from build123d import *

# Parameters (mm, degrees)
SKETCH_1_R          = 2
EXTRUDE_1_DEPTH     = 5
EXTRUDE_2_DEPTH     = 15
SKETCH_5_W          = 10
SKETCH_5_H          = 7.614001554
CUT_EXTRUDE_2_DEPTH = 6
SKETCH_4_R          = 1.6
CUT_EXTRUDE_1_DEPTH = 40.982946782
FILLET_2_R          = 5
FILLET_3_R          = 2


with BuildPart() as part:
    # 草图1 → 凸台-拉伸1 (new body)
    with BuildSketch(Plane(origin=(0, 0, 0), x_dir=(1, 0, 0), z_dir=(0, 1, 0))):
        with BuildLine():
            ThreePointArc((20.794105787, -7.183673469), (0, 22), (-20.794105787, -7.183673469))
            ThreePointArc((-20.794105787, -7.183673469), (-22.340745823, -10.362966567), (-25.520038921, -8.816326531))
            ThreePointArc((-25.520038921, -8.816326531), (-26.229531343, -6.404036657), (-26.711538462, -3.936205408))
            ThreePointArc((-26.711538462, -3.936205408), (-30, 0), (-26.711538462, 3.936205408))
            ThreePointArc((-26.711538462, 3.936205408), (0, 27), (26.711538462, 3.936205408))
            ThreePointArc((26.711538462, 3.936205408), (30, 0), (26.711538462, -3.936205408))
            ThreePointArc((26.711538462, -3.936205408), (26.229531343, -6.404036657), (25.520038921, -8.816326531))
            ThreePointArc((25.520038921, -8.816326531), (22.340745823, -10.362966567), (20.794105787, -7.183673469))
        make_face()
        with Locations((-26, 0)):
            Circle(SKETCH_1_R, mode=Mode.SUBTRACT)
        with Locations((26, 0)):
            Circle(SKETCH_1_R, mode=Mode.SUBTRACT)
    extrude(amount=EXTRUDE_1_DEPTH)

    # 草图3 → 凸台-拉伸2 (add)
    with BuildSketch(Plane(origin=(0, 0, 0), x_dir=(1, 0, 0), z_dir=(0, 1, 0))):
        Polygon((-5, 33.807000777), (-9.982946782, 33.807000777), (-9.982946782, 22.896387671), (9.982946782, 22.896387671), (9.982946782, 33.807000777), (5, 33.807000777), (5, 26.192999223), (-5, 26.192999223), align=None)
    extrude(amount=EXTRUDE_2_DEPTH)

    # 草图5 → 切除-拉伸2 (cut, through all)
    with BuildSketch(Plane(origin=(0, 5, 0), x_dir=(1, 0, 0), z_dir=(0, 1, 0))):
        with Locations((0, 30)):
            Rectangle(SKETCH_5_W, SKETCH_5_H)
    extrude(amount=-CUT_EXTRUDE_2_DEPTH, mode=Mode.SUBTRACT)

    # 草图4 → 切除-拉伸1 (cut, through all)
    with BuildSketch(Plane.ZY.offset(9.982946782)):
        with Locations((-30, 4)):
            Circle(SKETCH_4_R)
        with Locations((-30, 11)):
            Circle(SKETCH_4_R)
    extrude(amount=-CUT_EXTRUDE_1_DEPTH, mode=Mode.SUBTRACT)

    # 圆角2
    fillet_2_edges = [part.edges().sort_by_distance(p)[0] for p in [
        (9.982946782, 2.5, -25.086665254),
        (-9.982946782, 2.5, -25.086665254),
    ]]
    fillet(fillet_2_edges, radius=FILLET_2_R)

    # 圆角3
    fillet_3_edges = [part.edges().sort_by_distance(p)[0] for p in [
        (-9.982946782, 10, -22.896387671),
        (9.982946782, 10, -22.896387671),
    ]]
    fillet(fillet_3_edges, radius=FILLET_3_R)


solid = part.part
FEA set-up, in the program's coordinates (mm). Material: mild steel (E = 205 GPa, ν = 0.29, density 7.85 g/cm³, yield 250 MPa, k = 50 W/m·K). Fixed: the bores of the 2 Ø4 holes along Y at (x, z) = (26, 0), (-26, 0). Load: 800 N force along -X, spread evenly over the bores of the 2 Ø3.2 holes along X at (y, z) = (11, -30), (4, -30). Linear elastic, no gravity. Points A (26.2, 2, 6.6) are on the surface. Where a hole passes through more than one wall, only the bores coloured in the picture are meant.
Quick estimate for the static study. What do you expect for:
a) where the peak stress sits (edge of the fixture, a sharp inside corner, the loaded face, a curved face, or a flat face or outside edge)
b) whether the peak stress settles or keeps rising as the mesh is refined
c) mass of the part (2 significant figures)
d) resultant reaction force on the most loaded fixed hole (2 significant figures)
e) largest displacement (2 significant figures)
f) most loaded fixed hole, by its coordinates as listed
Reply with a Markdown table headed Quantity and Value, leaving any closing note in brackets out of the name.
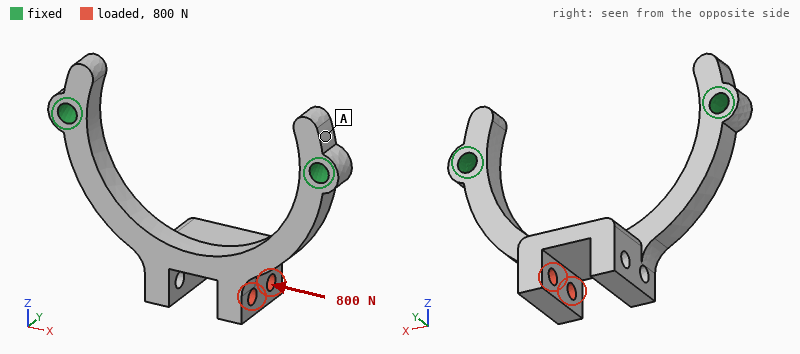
| Quantity | Value |
|---|---|
| where the peak stress sits | a sharp inside corner |
| whether the peak stress settles or keeps rising as the mesh is refined | keeps rising |
| mass of the part | 32 g |
| resultant reaction force on the most loaded fixed hole | 580 N |
| largest displacement | 38 µm |
| most loaded fixed hole, by its coordinates as listed | (-26, 0) |
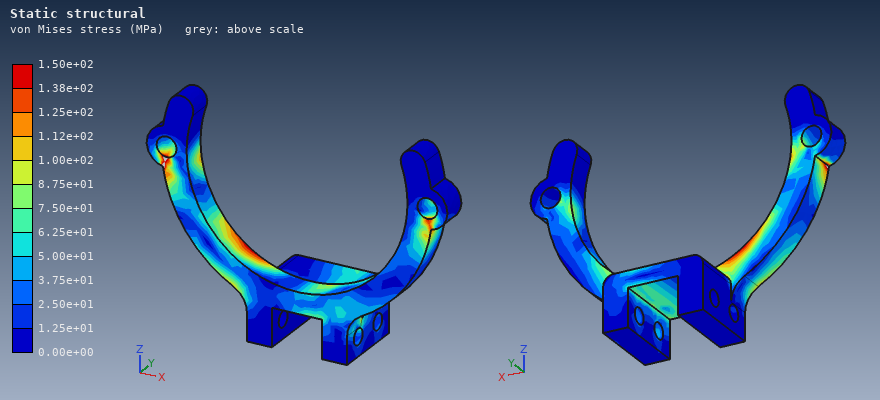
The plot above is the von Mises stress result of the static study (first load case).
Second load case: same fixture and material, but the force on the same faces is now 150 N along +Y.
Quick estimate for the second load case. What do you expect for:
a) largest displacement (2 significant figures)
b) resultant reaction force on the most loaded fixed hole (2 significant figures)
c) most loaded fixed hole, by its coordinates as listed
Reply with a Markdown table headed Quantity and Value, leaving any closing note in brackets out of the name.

| Quantity | Value |
|---|---|
| largest displacement | 0.10 mm |
| resultant reaction force on the most loaded fixed hole | 100 N |
| most loaded fixed hole, by its coordinates as listed | (26, 0) |
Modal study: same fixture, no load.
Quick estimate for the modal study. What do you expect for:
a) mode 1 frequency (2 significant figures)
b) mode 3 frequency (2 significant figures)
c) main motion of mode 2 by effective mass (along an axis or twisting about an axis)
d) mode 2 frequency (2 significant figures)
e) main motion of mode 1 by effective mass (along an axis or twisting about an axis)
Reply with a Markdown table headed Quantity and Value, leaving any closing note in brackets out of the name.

| Quantity | Value |
|---|---|
| mode 1 frequency | 1800 Hz |
| mode 3 frequency | 6800 Hz |
| main motion of mode 2 by effective mass | along X |
| mode 2 frequency | 5700 Hz |
| main motion of mode 1 by effective mass | along Y |
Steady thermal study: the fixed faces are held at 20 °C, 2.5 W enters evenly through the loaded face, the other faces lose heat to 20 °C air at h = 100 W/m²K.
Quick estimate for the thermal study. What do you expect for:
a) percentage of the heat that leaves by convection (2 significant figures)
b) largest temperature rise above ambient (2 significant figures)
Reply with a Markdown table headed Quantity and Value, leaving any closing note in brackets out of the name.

| Quantity | Value |
|---|---|
| percentage of the heat that leaves by convection | 75 % |
| largest temperature rise above ambient | 16 K |
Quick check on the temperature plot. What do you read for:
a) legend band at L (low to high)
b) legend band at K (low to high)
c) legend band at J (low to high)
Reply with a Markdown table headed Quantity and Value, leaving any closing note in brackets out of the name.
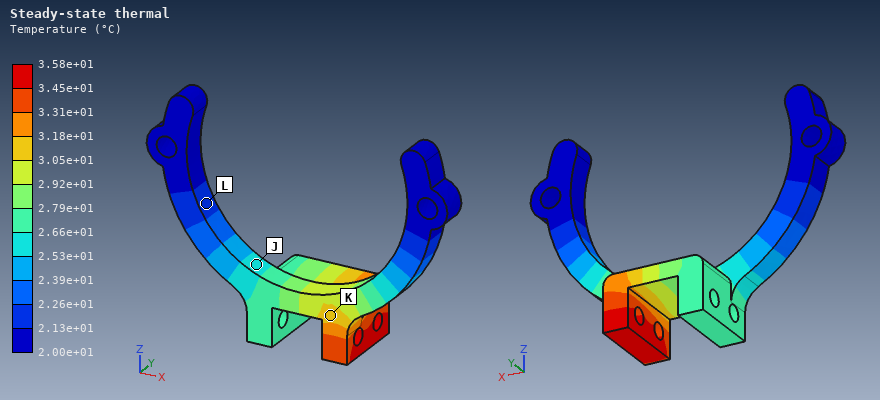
| Quantity | Value |
|---|---|
| legend band at L | 2.13e+01 to 2.26e+01 °C |
| legend band at K | 3.05e+01 to 3.18e+01 °C |
| legend band at J | 2.53e+01 to 2.66e+01 °C |
